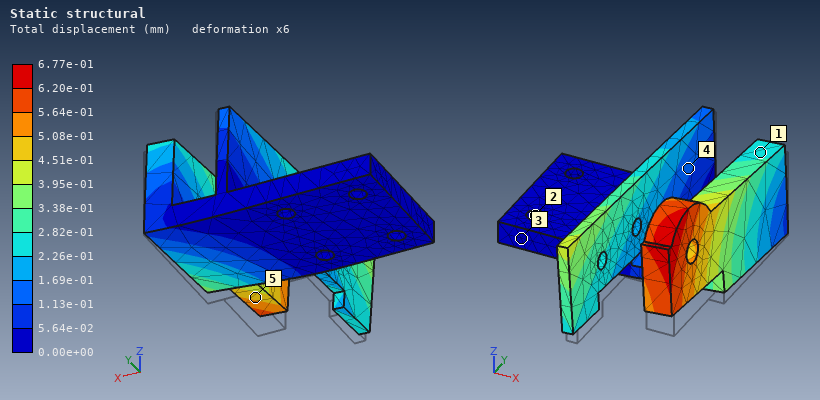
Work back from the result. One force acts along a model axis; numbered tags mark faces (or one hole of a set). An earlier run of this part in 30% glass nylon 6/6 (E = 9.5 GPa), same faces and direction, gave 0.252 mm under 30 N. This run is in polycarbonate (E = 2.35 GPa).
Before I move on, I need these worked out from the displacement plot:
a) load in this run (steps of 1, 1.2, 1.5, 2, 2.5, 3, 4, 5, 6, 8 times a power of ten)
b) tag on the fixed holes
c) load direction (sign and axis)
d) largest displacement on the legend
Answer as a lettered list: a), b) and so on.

a) 20 N
b) 2
c) +Z
d) 6.77e-01 mm
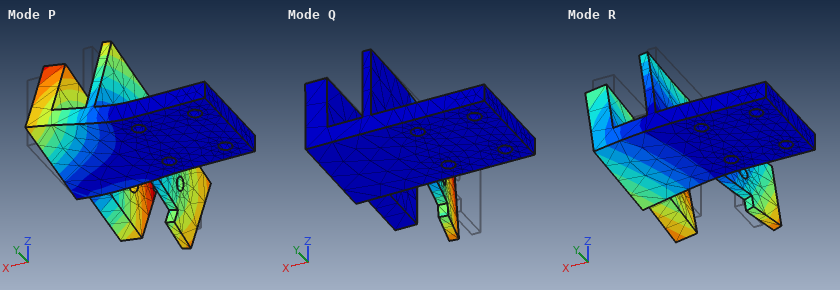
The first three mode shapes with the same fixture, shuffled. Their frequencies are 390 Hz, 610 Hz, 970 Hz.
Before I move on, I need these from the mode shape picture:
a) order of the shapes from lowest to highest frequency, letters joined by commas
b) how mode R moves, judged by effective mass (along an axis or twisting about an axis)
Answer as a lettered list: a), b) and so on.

a) Q, R, P
b) along Z
